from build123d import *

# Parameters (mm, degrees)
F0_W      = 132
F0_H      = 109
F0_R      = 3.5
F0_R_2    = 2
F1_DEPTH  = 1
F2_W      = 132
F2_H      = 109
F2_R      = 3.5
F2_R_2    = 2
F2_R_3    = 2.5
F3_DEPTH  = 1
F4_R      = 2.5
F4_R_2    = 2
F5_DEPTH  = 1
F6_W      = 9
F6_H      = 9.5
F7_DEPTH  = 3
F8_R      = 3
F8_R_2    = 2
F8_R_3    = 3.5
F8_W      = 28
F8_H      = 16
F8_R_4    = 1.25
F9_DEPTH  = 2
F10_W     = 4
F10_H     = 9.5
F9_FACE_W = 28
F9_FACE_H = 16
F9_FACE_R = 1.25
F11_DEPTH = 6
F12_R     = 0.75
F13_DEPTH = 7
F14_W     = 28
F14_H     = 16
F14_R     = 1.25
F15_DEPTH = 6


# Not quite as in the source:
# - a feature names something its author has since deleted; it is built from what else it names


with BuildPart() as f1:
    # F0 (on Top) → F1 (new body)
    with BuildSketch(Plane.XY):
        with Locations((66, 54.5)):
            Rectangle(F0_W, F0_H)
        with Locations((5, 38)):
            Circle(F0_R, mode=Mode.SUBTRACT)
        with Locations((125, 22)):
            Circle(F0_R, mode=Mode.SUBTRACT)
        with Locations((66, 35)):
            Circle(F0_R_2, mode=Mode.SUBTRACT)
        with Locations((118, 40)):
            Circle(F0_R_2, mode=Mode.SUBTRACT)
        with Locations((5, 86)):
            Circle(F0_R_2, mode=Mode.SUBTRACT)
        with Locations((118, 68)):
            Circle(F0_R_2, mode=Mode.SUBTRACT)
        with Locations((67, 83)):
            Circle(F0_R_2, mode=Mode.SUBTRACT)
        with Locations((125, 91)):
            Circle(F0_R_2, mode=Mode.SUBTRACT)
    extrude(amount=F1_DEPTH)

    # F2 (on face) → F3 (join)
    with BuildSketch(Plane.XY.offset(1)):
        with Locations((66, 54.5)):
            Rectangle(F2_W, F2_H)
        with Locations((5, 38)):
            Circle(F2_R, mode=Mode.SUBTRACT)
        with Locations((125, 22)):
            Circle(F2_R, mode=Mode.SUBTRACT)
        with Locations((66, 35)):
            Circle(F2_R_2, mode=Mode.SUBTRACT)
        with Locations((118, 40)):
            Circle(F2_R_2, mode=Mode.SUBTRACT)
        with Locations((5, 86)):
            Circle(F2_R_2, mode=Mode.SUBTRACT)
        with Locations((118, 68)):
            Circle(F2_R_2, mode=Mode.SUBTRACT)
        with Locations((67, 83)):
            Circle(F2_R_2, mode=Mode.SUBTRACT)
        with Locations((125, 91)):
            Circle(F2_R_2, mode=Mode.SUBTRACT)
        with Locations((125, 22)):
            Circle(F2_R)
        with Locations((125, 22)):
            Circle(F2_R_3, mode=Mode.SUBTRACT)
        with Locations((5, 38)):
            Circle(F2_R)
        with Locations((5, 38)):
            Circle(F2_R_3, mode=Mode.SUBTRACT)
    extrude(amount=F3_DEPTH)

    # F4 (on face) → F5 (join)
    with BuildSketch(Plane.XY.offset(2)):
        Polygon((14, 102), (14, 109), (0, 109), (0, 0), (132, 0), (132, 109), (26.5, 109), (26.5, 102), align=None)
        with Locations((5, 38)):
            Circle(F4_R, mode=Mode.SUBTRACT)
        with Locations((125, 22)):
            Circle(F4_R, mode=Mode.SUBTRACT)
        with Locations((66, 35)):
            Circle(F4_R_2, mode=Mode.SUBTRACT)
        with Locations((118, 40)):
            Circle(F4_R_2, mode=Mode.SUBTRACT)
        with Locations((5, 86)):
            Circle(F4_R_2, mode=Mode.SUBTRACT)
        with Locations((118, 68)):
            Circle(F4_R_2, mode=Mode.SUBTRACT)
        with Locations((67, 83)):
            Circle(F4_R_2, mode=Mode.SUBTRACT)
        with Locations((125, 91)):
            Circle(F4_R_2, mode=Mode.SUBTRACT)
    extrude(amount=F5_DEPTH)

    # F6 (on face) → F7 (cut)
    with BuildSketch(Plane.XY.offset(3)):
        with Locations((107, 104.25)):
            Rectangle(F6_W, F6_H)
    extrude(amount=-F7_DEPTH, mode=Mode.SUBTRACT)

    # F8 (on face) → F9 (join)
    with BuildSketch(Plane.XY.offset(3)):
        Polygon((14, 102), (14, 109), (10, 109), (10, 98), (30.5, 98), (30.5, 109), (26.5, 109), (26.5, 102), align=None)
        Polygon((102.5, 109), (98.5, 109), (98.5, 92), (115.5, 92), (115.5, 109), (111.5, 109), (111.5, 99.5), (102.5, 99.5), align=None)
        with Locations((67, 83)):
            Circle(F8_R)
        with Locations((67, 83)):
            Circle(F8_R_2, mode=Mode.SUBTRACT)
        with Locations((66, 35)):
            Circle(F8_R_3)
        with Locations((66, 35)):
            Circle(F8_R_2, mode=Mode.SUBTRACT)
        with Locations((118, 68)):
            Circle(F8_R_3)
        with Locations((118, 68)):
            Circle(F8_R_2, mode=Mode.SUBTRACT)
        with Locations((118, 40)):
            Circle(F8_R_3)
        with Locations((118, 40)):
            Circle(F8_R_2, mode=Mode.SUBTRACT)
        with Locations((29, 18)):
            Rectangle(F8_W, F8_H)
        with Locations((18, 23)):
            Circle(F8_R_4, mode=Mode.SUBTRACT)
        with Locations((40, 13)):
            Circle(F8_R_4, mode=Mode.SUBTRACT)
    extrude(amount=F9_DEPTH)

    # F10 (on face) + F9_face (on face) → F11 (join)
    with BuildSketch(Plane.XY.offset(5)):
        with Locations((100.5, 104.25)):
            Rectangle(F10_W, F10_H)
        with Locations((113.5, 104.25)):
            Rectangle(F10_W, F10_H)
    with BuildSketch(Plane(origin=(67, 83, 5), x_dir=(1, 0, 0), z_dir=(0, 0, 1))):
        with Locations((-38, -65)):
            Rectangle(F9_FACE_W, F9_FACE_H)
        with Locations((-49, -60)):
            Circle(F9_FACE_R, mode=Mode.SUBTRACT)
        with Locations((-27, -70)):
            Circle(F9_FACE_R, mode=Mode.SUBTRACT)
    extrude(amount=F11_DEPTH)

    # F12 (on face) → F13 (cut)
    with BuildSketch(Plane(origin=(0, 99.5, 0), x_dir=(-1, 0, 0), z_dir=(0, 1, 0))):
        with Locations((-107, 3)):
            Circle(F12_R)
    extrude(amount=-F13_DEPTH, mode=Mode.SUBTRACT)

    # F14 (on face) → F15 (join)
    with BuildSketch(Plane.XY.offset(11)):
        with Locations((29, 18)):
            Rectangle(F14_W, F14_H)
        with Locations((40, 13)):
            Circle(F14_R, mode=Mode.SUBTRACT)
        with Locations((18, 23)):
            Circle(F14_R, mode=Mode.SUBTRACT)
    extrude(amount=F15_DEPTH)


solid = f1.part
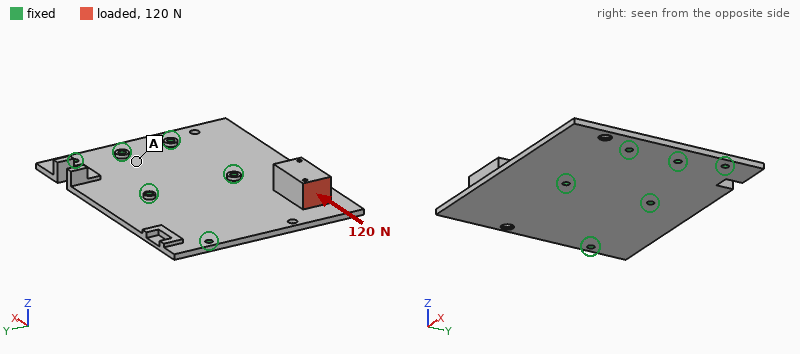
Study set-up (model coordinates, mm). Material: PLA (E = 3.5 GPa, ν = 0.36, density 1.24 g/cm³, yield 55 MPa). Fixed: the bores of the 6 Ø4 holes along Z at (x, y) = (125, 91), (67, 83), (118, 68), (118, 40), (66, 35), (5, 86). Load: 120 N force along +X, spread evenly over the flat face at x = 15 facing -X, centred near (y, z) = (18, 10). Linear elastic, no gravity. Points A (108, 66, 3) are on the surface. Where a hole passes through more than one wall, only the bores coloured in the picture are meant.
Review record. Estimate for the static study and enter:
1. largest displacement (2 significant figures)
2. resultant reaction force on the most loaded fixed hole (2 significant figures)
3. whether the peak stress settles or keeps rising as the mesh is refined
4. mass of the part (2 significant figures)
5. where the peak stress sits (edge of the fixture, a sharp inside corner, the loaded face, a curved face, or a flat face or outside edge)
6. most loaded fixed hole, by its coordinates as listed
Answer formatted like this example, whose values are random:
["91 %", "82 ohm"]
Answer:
["1.9 mm", "82 N", "keeps rising", "62 g", "edge of the fixture", "(66, 35)"]
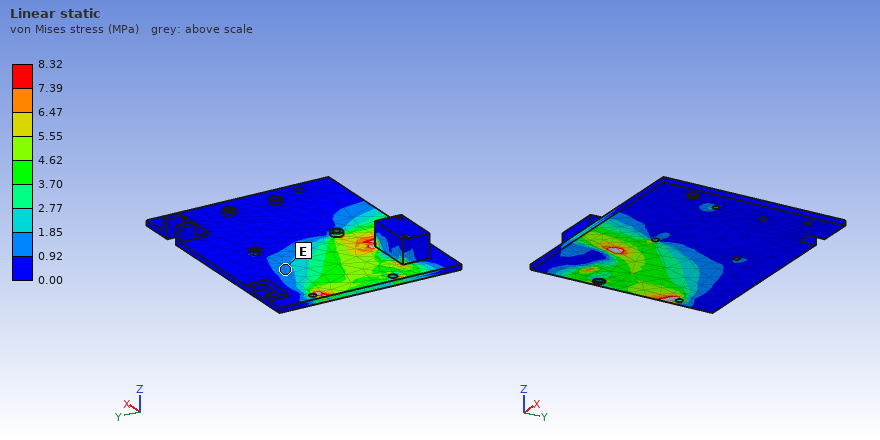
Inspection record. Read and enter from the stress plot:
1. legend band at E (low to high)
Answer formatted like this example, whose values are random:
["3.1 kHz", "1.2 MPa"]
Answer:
["0.92 to 1.85 MPa"]
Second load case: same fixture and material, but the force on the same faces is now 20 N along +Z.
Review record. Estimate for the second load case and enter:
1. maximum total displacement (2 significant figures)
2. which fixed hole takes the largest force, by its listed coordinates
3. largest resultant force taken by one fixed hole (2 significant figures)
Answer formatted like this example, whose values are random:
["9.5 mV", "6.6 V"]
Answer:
["1.8 mm", "(66, 35)", "23 N"]
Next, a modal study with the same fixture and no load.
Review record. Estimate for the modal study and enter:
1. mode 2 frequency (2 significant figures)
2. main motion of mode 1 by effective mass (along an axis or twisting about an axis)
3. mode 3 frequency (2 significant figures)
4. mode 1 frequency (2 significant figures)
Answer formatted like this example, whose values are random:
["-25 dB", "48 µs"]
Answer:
["540 Hz", "along Z", "670 Hz", "210 Hz"]
